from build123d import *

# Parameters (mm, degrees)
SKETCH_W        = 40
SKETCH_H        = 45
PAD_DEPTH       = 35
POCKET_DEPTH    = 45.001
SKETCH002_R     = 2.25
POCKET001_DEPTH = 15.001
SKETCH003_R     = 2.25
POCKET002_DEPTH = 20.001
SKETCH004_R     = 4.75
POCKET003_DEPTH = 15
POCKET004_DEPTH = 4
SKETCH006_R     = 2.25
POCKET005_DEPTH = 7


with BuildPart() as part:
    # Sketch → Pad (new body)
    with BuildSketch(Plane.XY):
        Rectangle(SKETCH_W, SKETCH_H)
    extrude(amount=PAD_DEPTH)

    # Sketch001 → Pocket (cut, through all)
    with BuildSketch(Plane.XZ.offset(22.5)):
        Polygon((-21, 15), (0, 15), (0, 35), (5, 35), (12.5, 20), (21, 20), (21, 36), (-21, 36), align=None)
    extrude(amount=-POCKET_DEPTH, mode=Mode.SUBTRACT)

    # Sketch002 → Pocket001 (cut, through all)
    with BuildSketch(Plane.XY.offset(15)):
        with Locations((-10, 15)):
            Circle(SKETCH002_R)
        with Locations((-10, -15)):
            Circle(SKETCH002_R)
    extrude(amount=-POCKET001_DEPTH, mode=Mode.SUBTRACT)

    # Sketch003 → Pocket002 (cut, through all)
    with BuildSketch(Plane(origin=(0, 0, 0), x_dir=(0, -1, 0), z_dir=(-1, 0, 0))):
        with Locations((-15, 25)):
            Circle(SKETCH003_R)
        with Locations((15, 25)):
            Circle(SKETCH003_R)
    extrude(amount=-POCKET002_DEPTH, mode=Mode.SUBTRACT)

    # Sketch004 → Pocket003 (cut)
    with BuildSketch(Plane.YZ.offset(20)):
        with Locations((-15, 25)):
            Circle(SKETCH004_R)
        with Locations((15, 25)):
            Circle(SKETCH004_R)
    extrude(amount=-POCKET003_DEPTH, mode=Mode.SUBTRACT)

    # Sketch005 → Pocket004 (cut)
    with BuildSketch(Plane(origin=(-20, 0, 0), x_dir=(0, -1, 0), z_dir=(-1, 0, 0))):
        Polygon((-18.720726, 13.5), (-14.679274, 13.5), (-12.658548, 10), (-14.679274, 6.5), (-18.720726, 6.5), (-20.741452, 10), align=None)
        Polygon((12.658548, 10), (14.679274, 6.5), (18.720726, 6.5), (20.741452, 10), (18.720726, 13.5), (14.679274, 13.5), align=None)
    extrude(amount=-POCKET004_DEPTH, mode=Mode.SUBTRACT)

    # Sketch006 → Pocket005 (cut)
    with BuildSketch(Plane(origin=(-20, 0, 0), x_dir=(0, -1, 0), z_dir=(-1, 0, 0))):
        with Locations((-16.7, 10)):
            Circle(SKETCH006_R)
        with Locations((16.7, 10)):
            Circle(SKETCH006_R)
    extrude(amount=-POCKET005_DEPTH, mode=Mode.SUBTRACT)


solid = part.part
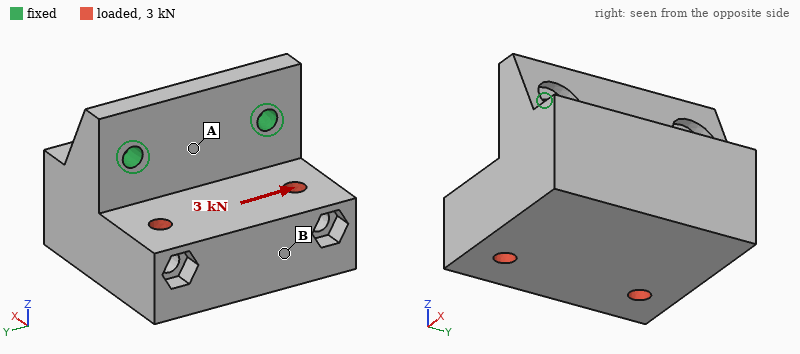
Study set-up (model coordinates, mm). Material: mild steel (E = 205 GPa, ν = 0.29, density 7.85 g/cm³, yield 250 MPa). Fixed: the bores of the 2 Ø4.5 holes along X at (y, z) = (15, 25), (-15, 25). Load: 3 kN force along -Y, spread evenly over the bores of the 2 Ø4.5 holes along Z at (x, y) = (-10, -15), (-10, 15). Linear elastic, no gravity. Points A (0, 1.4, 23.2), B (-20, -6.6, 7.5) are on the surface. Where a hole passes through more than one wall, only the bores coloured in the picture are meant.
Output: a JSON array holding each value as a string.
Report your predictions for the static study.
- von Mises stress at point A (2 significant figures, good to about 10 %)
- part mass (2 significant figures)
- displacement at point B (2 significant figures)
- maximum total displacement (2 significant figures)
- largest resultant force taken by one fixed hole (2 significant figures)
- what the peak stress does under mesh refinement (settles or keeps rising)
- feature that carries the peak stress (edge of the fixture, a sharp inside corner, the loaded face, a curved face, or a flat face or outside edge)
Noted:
["23 MPa", "280 g", "9.3 µm", "11 µm", "2.5 kN", "keeps rising", "edge of the fixture"]
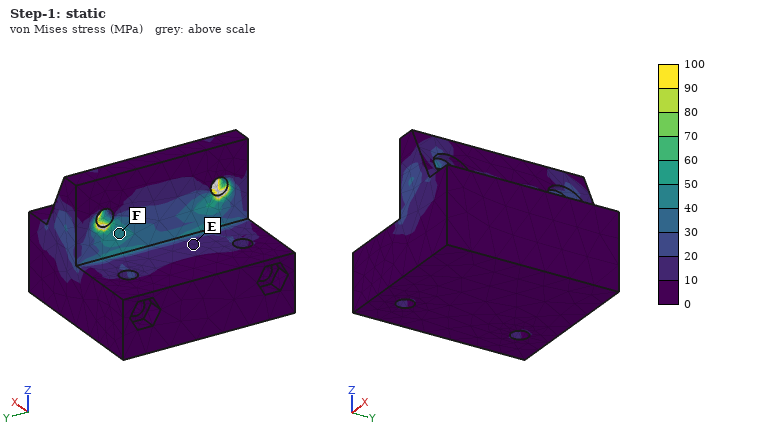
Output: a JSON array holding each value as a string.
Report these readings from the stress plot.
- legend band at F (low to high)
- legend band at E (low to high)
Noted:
["40 to 50 MPa", "10 to 20 MPa"]
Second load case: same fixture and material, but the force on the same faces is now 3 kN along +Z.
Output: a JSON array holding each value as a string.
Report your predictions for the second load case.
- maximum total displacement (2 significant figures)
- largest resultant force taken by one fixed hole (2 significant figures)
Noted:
["50 µm", "1.5 kN"]
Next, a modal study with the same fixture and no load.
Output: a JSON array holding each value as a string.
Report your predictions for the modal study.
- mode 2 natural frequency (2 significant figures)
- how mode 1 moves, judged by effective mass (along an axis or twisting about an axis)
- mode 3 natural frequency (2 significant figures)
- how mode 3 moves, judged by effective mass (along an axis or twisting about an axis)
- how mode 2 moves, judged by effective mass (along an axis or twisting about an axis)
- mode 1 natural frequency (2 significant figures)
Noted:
["8200 Hz", "along X", "12 kHz", "along Y", "along Y", "2800 Hz"]
